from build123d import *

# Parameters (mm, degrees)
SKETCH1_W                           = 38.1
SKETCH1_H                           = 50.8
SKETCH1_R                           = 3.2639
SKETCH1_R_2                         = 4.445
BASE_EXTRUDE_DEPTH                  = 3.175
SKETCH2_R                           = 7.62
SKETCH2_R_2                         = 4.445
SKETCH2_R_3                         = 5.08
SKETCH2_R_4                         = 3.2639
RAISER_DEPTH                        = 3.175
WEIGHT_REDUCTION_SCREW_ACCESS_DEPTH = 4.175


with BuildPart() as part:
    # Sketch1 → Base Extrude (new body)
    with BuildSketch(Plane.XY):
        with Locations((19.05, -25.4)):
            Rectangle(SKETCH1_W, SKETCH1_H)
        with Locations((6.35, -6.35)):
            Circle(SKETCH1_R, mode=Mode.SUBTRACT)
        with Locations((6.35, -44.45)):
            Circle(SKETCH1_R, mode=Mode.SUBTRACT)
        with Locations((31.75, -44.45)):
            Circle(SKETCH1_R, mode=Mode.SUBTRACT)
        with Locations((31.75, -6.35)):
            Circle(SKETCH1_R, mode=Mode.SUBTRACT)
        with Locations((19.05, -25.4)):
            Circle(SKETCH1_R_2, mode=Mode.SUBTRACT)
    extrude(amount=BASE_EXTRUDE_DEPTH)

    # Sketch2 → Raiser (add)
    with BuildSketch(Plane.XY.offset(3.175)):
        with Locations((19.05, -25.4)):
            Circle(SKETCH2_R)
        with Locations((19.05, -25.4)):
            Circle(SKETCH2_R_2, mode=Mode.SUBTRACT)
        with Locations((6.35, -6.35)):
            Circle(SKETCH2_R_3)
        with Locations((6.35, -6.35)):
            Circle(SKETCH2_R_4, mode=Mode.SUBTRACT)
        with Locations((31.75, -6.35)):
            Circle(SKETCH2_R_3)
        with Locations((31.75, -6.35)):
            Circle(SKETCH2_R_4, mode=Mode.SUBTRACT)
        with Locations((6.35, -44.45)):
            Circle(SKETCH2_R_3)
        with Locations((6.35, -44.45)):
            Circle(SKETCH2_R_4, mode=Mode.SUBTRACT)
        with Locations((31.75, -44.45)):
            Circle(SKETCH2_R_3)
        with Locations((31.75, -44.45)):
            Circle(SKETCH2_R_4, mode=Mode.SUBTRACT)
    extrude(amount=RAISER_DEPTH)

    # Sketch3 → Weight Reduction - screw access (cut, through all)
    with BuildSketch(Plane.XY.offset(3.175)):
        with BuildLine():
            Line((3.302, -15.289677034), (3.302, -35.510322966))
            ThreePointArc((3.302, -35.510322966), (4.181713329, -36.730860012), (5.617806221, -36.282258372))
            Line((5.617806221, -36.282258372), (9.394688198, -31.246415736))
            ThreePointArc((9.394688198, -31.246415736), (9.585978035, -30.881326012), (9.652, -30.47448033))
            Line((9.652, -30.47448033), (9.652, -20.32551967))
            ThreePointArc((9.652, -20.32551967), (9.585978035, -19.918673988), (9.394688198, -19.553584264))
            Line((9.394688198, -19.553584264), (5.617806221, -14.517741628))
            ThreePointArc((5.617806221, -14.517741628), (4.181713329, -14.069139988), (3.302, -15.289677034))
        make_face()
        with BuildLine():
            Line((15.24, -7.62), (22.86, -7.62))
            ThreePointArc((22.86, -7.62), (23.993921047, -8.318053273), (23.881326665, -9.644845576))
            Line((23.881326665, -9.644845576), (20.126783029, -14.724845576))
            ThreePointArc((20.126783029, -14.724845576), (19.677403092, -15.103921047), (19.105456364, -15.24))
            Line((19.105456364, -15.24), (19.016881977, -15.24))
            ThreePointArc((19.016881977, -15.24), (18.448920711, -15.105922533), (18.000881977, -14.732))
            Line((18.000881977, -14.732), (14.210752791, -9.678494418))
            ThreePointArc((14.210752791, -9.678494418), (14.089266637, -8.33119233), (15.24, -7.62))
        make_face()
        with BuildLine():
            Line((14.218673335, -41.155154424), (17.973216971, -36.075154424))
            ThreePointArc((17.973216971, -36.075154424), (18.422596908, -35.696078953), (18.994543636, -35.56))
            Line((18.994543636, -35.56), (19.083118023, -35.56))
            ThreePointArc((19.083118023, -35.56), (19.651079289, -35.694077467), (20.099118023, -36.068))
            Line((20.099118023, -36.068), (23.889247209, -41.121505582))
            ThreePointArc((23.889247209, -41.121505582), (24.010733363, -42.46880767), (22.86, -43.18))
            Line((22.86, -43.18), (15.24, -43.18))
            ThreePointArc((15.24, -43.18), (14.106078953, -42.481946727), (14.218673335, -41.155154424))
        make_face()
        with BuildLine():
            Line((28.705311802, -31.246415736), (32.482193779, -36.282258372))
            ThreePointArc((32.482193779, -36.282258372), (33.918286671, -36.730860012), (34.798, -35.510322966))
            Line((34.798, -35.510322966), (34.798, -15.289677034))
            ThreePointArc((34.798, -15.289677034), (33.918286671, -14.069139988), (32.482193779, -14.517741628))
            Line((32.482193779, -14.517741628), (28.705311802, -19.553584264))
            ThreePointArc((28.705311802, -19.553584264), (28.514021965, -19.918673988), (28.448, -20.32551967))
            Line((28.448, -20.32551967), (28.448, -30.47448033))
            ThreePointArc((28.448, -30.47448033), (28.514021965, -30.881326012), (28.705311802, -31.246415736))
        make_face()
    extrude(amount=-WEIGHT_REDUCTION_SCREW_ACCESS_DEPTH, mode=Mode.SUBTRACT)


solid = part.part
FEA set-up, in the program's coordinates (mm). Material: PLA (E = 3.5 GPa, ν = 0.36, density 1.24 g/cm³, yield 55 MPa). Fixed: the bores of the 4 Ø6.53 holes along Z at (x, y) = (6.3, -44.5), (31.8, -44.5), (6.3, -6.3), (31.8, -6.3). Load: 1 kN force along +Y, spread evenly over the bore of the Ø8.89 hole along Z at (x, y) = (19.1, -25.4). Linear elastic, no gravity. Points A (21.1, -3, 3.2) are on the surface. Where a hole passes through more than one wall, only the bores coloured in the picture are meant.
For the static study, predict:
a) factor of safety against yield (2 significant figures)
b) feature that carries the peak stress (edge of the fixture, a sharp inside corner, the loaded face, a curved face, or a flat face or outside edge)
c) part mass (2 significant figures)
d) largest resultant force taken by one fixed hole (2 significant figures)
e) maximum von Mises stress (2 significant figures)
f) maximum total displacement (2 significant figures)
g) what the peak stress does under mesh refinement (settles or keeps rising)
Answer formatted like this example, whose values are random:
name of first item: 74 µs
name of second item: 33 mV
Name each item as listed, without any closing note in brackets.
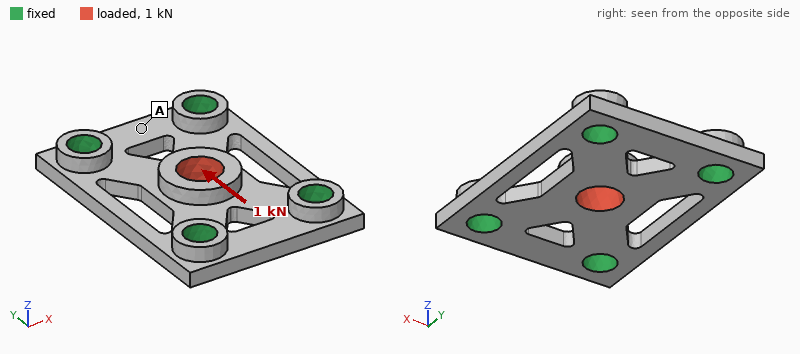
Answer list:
factor of safety against yield: 2.0
feature that carries the peak stress: a curved face
part mass: 6.7 g
largest resultant force taken by one fixed hole: 280 N
maximum von Mises stress: 28 MPa
maximum total displacement: 99 µm
what the peak stress does under mesh refinement: settles
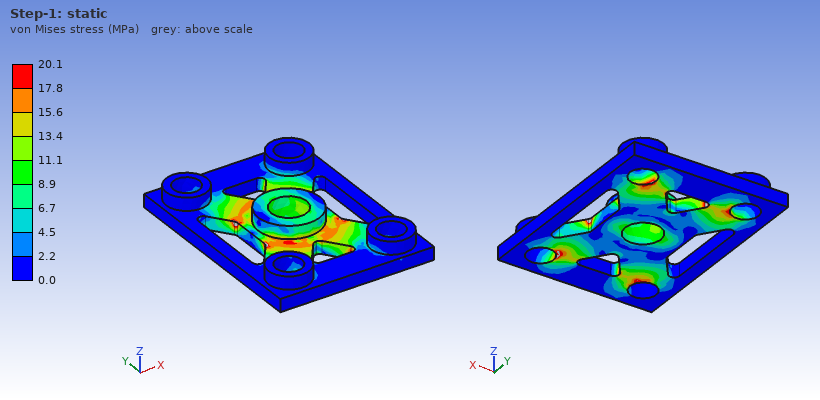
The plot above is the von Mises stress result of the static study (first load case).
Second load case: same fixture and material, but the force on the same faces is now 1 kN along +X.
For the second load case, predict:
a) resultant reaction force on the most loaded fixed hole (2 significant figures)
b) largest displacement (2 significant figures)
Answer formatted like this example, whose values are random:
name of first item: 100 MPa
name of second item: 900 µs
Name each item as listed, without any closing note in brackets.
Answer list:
resultant reaction force on the most loaded fixed hole: 320 N
largest displacement: 0.19 mm
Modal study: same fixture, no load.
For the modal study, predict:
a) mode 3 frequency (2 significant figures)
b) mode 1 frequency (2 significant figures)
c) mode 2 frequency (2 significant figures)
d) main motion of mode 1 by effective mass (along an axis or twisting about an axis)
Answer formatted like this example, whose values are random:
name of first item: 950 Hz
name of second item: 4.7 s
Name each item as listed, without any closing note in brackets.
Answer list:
mode 3 frequency: 5800 Hz
mode 1 frequency: 4700 Hz
mode 2 frequency: 5800 Hz
main motion of mode 1 by effective mass: along Z
